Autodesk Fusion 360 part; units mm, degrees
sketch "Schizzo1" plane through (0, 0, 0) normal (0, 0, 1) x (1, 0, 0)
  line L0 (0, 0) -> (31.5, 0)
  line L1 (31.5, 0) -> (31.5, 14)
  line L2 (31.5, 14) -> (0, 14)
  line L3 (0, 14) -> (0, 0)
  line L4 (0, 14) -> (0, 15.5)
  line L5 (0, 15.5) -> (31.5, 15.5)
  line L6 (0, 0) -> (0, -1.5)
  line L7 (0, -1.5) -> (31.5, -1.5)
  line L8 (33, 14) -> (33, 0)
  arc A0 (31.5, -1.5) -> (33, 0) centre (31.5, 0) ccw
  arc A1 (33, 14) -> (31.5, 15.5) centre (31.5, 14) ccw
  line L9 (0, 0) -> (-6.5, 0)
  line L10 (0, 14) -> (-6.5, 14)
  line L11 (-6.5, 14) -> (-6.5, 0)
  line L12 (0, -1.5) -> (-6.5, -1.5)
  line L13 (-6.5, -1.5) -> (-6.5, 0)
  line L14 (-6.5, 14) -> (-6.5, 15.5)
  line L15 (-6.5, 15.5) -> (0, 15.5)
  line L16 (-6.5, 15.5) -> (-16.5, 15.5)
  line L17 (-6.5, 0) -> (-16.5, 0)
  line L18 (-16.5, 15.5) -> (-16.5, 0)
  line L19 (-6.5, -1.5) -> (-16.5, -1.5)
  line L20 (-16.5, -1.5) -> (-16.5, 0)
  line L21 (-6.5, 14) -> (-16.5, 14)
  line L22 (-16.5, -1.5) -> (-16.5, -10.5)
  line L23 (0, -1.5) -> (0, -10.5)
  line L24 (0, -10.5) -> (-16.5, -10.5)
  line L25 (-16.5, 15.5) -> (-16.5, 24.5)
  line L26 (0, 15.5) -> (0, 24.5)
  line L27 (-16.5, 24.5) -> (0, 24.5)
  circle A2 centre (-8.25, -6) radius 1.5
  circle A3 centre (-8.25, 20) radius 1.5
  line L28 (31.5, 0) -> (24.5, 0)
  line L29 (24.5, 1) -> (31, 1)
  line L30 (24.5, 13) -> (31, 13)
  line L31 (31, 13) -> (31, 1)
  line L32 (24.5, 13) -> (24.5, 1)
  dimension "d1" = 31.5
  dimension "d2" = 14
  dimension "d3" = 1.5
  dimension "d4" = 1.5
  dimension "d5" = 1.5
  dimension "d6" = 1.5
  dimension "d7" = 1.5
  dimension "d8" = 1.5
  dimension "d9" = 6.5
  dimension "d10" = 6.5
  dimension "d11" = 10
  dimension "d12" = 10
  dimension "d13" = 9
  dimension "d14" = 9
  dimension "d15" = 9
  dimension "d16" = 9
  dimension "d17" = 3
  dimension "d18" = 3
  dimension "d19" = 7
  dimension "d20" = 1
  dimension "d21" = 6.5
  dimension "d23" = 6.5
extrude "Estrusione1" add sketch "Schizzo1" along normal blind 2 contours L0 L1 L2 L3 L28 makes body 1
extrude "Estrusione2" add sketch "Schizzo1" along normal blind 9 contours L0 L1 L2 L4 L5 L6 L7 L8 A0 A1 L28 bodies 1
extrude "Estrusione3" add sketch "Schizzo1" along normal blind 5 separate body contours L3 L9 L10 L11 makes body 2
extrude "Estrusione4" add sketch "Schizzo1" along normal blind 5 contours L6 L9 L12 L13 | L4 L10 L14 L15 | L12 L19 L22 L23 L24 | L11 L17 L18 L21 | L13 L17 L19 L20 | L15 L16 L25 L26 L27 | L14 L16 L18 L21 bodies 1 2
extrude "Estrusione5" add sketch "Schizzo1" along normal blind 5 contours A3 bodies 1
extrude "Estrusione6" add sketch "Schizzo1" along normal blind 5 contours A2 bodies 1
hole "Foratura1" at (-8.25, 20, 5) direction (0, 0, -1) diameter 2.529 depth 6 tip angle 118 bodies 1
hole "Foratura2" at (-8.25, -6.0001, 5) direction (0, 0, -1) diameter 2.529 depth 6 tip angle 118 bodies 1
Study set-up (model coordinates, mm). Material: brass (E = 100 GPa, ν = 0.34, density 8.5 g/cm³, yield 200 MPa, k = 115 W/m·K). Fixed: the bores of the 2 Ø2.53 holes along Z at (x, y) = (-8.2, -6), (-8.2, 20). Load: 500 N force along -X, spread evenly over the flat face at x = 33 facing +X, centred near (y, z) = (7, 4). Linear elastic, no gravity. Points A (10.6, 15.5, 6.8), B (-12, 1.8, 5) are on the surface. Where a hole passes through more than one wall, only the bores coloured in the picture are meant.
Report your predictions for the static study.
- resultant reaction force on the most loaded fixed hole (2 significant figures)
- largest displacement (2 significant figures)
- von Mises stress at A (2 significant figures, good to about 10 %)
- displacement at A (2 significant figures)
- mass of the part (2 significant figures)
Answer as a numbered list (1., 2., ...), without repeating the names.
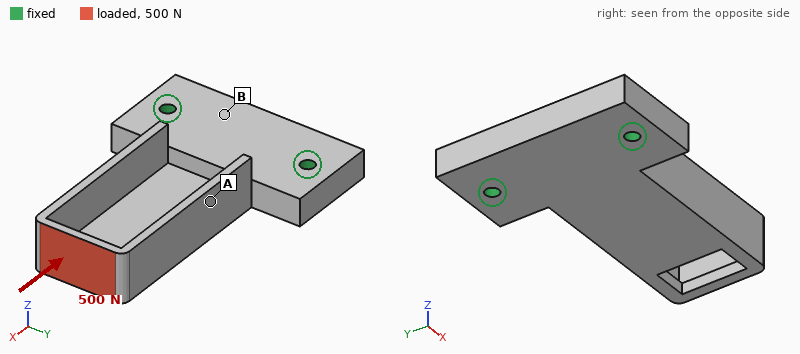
1. 260 N
2. 75 µm
3. 22 MPa
4. 17 µm
5. 39 g
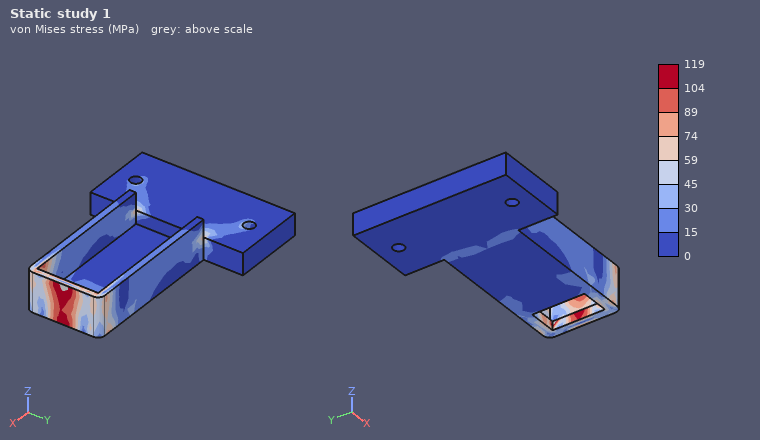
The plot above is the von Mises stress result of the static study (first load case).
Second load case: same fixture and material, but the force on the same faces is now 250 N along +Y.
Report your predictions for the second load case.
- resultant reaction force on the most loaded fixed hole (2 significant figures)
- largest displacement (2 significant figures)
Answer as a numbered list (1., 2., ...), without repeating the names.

1. 420 N
2. 0.18 mm
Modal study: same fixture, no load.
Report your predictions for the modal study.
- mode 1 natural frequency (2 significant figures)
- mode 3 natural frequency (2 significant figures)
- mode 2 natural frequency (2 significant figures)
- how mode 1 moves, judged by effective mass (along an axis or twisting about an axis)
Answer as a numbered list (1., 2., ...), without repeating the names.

1. 1800 Hz
2. 6000 Hz
3. 2700 Hz
4. along Z
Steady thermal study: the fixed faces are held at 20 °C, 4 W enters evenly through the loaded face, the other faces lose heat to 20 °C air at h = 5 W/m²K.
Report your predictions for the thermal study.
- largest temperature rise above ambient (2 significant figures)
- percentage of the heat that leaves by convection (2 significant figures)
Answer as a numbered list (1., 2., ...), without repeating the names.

1. 33 K
2. 4.5 %
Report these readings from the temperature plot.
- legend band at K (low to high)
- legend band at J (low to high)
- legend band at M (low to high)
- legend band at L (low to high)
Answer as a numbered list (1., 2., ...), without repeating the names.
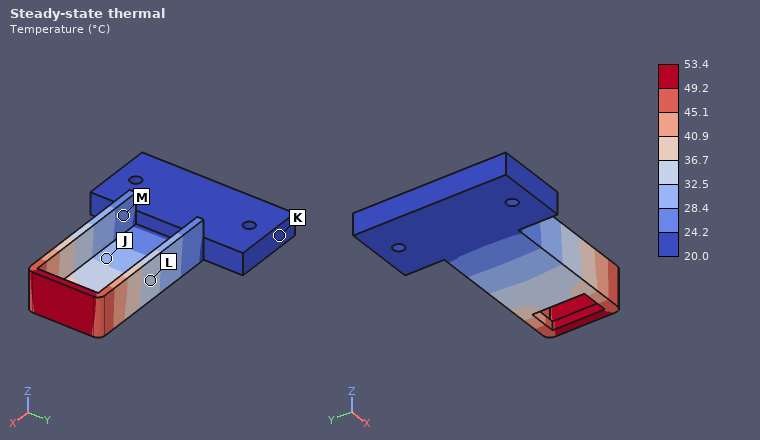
1. 20.0 to 24.2 °C
2. 28.4 to 32.5 °C
3. 24.2 to 28.4 °C
4. 32.5 to 36.7 °C
